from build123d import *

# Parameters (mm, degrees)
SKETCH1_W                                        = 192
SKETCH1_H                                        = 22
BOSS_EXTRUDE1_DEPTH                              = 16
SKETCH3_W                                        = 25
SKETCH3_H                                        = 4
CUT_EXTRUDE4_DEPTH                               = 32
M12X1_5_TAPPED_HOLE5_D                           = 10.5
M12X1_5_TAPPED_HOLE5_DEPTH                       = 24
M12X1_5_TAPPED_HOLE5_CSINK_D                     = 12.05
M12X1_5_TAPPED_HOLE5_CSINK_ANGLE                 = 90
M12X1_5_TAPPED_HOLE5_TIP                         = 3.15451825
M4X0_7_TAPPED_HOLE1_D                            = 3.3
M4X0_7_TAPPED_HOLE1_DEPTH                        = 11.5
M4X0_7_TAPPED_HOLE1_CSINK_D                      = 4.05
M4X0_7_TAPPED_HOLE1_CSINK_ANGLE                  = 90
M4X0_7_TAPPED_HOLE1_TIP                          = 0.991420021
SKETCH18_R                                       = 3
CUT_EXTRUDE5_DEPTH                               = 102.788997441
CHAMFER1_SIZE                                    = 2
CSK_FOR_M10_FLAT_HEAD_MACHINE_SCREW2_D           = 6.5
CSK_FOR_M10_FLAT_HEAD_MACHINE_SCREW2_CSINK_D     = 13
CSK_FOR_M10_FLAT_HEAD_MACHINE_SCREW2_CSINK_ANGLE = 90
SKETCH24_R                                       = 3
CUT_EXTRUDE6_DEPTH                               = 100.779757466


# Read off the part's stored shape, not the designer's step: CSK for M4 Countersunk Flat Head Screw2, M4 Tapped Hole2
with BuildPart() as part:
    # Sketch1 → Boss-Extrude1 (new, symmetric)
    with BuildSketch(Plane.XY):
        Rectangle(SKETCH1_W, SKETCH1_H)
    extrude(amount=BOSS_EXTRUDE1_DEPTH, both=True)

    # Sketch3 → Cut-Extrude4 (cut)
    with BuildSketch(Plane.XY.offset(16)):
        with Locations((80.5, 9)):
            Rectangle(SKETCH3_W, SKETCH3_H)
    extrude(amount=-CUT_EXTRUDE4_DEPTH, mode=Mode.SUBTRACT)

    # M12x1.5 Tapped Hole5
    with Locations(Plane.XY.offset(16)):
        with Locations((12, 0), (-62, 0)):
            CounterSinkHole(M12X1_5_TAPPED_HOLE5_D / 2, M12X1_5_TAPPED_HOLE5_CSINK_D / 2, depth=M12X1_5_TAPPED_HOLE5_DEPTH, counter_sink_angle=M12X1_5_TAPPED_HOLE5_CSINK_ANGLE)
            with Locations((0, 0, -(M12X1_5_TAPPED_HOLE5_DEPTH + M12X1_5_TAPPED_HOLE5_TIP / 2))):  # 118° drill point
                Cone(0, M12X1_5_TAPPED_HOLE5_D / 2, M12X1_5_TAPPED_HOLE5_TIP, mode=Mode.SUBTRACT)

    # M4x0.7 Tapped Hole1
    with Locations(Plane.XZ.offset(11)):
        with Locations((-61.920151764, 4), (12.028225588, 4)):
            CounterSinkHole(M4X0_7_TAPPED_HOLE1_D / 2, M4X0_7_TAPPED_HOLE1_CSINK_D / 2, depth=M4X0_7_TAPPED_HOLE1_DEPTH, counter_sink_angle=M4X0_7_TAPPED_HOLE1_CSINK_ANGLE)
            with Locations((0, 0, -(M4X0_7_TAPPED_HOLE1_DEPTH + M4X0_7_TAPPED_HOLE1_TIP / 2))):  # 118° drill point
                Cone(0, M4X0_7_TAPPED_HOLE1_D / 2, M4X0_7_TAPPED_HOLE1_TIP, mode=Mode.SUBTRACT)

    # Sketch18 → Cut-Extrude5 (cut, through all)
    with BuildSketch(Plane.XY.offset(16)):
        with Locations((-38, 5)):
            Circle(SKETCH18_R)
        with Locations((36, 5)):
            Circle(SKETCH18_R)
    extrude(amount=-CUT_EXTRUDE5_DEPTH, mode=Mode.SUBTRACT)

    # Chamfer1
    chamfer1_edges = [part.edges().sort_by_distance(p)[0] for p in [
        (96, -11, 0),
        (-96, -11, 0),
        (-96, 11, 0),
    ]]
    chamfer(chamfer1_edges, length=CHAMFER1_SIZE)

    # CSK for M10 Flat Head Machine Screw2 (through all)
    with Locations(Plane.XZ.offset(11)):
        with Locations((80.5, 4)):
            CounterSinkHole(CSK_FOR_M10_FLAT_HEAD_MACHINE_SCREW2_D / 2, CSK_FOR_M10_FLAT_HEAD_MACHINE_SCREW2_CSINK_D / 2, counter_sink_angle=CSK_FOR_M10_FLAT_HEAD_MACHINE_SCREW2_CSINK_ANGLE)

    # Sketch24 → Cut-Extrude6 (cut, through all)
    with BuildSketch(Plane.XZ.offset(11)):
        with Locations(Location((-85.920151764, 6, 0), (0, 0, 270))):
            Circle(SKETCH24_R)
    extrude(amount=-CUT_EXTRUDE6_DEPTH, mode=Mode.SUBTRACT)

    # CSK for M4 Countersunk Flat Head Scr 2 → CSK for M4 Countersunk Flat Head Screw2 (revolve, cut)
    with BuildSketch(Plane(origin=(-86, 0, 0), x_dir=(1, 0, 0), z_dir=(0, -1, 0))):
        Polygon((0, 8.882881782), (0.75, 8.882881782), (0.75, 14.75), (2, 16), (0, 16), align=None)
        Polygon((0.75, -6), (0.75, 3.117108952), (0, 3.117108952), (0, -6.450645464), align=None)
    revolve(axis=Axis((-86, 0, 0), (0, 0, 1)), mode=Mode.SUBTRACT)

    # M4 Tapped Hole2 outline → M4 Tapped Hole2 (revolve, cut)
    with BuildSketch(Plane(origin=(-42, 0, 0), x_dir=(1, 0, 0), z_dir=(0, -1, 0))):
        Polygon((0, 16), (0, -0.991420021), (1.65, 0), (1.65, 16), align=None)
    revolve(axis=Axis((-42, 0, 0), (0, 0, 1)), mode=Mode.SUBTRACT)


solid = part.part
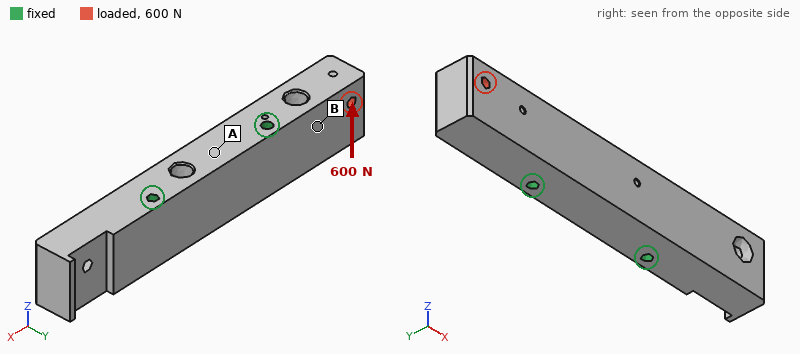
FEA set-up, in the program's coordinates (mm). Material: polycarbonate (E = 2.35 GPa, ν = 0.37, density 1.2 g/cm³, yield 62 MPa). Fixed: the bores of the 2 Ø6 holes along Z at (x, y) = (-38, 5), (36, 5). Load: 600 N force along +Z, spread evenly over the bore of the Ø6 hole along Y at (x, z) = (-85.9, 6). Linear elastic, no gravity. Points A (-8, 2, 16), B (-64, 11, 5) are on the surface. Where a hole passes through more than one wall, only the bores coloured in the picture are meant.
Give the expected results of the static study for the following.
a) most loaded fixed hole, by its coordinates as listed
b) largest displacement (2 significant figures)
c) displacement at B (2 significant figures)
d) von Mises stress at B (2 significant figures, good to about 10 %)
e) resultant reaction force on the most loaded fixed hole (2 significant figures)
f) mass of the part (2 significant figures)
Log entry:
(-38, 5)
0.35 mm
0.10 mm
3.6 MPa
660 N
150 g
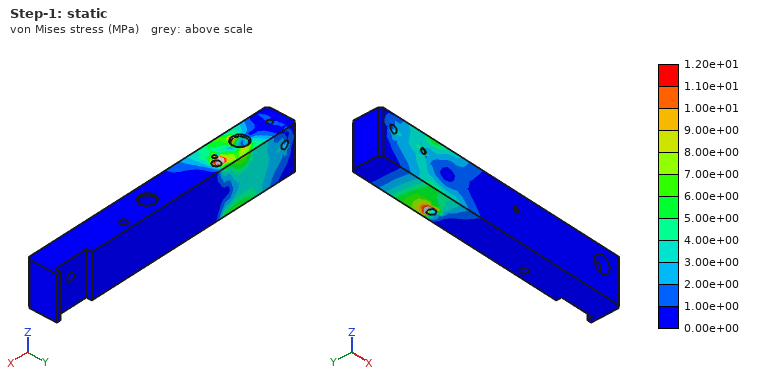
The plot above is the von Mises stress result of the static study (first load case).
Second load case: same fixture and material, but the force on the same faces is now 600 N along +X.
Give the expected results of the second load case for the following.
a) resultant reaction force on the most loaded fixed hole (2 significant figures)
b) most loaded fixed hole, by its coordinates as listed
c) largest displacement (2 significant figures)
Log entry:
530 N
(-38, 5)
86 µm
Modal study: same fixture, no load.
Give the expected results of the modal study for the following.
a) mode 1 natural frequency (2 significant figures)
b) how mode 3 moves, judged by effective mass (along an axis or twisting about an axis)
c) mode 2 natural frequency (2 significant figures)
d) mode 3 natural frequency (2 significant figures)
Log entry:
1100 Hz
along Z
1100 Hz
1600 Hz
